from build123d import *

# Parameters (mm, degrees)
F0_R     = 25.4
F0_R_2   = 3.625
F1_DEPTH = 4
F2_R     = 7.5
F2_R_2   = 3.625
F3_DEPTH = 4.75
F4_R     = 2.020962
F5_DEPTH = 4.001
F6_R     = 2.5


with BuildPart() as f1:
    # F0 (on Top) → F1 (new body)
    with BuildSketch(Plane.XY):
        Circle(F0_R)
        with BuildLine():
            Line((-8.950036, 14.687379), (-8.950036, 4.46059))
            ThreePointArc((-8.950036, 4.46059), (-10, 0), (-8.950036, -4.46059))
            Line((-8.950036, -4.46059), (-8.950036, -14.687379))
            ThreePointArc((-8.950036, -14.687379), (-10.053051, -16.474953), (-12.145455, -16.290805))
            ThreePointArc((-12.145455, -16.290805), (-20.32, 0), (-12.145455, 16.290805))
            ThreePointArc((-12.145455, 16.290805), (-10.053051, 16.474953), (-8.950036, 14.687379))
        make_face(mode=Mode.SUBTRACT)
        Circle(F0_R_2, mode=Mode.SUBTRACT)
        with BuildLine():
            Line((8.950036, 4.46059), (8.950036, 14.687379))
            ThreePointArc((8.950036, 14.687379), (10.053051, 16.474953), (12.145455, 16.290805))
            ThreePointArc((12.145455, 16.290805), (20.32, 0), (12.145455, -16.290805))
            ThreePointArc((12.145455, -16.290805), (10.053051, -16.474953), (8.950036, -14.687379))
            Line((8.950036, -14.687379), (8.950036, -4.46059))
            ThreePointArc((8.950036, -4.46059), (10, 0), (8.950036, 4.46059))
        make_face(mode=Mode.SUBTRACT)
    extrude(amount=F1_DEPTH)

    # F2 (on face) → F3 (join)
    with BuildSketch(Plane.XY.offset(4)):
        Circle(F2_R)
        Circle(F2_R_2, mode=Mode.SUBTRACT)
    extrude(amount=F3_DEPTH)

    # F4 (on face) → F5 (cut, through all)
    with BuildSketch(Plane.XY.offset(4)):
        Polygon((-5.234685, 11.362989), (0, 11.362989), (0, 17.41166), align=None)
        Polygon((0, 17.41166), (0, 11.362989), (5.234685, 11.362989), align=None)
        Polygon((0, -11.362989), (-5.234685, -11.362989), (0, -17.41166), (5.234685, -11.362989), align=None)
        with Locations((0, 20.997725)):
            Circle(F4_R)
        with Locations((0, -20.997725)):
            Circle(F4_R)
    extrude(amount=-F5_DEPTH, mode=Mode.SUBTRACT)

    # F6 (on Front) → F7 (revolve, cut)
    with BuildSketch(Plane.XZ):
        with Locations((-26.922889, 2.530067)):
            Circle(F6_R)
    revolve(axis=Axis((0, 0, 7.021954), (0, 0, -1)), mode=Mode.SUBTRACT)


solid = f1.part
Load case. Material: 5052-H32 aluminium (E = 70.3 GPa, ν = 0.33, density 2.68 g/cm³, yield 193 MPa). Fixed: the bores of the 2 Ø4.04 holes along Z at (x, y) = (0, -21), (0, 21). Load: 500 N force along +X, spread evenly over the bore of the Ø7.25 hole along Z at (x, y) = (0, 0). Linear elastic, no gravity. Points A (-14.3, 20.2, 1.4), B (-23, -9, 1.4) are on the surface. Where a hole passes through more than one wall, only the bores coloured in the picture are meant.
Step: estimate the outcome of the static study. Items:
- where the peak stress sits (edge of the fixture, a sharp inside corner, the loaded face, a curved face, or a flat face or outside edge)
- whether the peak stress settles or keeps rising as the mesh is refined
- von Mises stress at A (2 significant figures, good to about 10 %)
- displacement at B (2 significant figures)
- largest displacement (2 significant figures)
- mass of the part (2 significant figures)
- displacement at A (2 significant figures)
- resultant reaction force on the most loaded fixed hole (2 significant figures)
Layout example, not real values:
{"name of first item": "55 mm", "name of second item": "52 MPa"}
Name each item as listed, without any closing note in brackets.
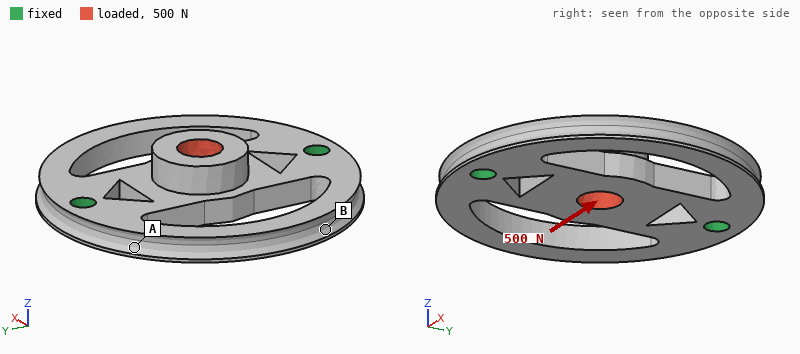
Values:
{"where the peak stress sits": "edge of the fixture", "whether the peak stress settles or keeps rising as the mesh is refined": "keeps rising", "von Mises stress at A": "8.1 MPa", "displacement at B": "8.7 µm", "largest displacement": "17 µm", "mass of the part": "15 g", "displacement at A": "3.9 µm", "resultant reaction force on the most loaded fixed hole": "250 N"}
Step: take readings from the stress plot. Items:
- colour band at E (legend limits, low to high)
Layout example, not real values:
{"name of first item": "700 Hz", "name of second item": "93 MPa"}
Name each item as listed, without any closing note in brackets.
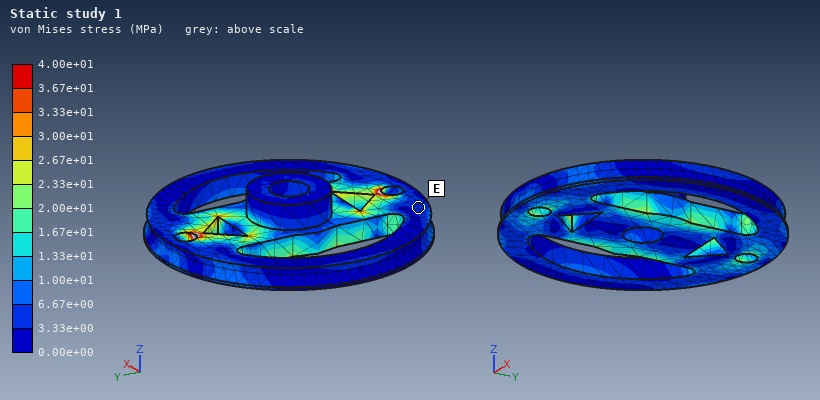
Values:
{"colour band at E": "3.33e+00 to 6.67e+00 MPa"}
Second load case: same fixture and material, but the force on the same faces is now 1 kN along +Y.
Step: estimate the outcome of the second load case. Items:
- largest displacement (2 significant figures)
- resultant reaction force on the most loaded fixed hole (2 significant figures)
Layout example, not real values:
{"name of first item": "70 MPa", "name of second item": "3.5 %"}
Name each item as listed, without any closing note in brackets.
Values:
{"largest displacement": "9.4 µm", "resultant reaction force on the most loaded fixed hole": "510 N"}
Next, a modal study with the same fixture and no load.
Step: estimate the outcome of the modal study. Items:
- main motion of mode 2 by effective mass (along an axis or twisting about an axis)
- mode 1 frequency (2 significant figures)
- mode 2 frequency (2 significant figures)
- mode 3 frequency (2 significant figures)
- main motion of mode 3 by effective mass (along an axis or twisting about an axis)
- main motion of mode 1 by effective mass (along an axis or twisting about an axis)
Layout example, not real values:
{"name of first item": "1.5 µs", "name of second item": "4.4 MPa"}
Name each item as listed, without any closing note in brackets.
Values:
{"main motion of mode 2 by effective mass": "along Z", "mode 1 frequency": "4600 Hz", "mode 2 frequency": "4900 Hz", "mode 3 frequency": "10 kHz", "main motion of mode 3 by effective mass": "along Z", "main motion of mode 1 by effective mass": "twisting about Y"}
